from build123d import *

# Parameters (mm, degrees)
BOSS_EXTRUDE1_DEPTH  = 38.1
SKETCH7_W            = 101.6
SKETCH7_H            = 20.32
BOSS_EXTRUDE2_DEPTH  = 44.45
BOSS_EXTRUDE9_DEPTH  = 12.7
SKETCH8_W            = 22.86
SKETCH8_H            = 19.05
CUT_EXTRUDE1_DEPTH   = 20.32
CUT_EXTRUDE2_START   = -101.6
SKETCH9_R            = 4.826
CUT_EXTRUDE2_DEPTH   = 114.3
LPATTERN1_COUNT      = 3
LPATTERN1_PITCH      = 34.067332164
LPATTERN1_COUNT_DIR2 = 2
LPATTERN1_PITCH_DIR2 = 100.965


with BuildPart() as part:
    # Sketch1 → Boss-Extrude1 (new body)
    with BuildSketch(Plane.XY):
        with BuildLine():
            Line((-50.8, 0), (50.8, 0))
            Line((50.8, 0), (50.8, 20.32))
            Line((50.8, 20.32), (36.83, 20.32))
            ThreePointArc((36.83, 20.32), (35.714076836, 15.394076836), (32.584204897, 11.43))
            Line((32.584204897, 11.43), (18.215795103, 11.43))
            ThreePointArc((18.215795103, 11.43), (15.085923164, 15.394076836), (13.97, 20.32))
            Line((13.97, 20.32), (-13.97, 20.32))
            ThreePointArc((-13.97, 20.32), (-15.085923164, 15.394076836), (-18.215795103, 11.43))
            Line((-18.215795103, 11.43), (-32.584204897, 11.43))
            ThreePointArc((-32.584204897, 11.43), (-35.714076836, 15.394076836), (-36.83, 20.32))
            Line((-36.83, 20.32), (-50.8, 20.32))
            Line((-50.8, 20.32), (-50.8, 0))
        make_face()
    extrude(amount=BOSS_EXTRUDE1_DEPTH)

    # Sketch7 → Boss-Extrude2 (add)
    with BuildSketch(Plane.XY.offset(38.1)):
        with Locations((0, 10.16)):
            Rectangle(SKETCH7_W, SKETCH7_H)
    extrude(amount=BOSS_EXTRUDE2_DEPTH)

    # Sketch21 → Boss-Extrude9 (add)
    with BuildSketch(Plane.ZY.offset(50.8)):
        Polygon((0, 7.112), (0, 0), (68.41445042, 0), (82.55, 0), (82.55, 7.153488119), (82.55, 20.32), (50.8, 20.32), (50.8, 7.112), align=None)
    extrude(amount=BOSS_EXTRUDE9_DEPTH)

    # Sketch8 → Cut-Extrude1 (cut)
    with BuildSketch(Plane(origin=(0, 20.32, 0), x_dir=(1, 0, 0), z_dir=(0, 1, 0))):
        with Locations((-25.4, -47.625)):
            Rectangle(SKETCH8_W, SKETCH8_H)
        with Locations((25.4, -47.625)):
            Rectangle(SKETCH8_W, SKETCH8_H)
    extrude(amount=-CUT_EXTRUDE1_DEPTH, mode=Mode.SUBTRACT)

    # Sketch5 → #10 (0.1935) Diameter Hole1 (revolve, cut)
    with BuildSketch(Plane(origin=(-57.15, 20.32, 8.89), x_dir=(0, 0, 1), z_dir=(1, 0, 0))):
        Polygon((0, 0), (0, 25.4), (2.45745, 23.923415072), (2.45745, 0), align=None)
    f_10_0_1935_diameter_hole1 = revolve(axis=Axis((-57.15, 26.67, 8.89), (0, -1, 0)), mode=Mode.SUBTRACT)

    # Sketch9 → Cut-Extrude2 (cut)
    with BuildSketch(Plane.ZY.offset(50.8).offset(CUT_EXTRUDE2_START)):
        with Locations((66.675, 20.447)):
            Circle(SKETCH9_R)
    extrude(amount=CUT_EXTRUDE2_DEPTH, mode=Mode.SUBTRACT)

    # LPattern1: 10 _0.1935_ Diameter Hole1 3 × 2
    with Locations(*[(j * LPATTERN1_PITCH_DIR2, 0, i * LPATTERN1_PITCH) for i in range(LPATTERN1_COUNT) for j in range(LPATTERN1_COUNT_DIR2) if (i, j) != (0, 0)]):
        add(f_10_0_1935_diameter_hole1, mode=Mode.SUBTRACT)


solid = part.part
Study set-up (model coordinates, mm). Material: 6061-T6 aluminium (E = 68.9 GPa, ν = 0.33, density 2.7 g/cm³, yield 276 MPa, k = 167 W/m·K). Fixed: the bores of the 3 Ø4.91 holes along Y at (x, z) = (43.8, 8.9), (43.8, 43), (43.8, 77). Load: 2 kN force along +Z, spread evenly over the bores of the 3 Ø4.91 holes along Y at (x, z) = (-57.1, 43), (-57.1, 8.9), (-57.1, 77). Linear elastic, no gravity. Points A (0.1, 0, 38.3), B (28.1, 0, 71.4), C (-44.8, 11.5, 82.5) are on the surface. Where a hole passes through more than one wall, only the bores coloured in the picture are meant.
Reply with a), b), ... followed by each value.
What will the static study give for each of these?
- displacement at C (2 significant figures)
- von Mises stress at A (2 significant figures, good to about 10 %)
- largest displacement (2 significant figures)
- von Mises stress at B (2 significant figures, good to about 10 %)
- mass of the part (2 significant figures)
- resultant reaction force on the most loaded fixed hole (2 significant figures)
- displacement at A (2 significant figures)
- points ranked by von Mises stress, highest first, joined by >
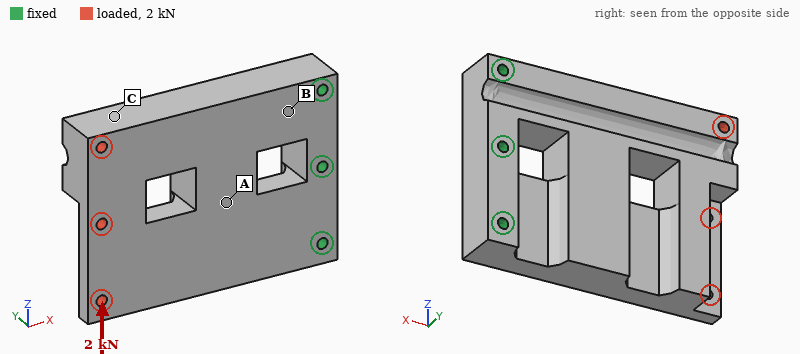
a) 33 µm
b) 6.1 MPa
c) 44 µm
d) 11 MPa
e) 390 g
f) 3.0 kN
g) 12 µm
h) B > A > C
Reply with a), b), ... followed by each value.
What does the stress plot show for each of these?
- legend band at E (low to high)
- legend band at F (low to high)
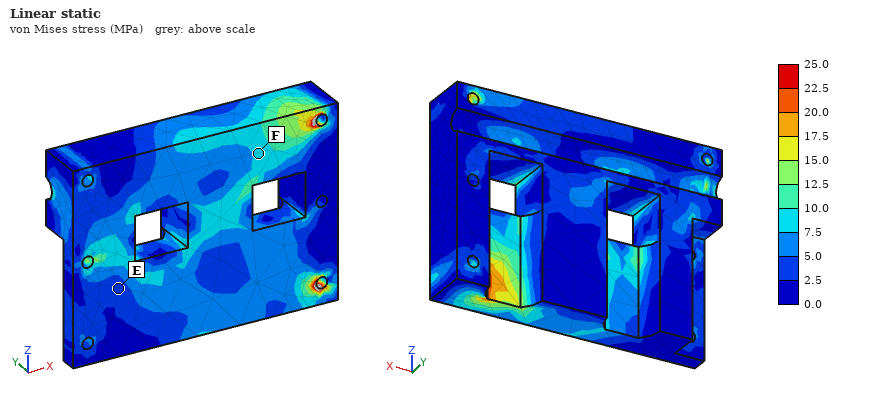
a) 2.5 to 5.0 MPa
b) 7.5 to 10.0 MPa
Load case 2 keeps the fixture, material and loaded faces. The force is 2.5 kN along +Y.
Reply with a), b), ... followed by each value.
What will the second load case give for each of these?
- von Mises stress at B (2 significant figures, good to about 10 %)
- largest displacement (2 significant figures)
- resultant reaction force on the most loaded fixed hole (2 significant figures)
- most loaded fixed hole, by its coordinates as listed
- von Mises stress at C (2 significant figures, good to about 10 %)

a) 89 MPa
b) 0.65 mm
c) 1.8 kN
d) (43.8, 77)
e) 18 MPa
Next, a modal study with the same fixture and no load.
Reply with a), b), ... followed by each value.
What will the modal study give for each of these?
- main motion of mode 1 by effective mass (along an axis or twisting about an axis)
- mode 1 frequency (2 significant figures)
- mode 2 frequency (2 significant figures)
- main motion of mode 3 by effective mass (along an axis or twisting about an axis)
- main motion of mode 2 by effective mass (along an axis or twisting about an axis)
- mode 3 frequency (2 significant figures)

a) along Y
b) 1000 Hz
c) 2900 Hz
d) along Z
e) twisting about X
f) 3700 Hz
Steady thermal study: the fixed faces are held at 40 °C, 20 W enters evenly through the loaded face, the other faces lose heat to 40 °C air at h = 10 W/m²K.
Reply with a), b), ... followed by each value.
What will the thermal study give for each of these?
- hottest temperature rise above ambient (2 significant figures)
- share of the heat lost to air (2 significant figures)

a) 14 K
b) 7.9 %
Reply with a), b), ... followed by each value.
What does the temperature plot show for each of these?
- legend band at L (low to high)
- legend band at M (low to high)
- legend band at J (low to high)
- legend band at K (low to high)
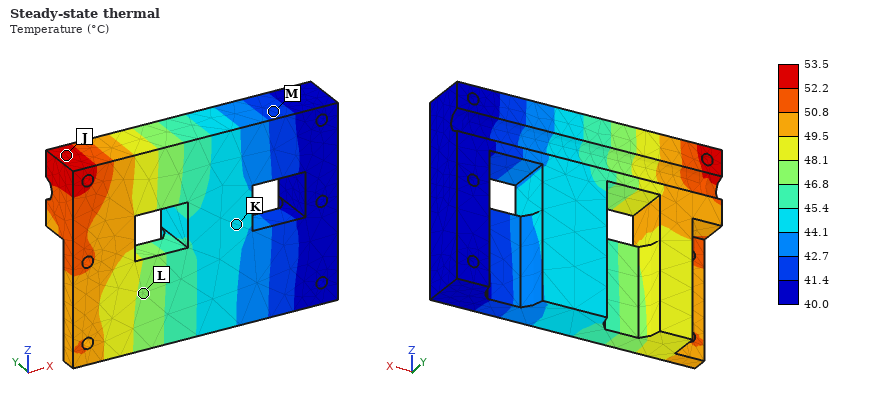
a) 46.8 to 48.1 °C
b) 41.4 to 42.7 °C
c) 52.2 to 53.5 °C
d) 44.1 to 45.4 °C
